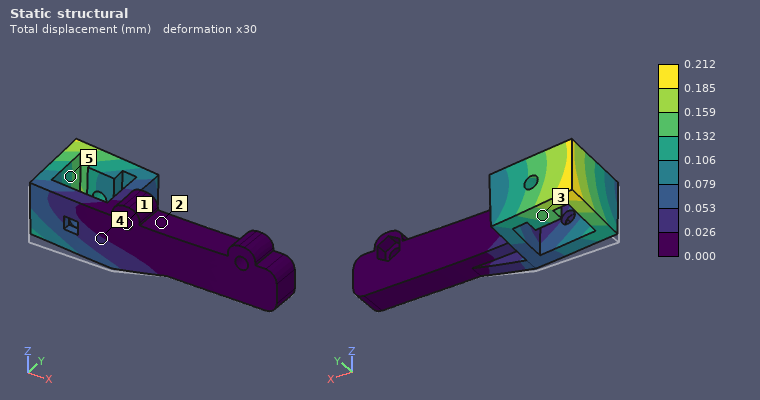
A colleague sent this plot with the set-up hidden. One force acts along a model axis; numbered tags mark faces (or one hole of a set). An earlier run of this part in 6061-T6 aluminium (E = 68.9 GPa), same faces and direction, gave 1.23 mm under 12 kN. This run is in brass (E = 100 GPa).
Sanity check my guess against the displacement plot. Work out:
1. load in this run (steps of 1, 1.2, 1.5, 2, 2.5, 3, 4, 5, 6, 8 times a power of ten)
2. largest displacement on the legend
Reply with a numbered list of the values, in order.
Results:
1. 3 kN
2. 0.212 mm
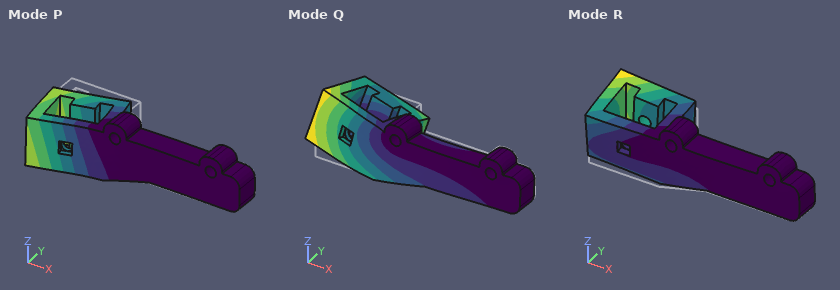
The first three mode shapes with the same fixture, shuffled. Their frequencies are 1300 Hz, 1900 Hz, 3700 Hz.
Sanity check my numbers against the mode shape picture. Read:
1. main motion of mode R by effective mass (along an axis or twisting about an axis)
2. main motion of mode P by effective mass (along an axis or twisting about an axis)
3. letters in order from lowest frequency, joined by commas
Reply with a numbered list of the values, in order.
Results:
1. along Z
2. along Y
3. P, R, Q
